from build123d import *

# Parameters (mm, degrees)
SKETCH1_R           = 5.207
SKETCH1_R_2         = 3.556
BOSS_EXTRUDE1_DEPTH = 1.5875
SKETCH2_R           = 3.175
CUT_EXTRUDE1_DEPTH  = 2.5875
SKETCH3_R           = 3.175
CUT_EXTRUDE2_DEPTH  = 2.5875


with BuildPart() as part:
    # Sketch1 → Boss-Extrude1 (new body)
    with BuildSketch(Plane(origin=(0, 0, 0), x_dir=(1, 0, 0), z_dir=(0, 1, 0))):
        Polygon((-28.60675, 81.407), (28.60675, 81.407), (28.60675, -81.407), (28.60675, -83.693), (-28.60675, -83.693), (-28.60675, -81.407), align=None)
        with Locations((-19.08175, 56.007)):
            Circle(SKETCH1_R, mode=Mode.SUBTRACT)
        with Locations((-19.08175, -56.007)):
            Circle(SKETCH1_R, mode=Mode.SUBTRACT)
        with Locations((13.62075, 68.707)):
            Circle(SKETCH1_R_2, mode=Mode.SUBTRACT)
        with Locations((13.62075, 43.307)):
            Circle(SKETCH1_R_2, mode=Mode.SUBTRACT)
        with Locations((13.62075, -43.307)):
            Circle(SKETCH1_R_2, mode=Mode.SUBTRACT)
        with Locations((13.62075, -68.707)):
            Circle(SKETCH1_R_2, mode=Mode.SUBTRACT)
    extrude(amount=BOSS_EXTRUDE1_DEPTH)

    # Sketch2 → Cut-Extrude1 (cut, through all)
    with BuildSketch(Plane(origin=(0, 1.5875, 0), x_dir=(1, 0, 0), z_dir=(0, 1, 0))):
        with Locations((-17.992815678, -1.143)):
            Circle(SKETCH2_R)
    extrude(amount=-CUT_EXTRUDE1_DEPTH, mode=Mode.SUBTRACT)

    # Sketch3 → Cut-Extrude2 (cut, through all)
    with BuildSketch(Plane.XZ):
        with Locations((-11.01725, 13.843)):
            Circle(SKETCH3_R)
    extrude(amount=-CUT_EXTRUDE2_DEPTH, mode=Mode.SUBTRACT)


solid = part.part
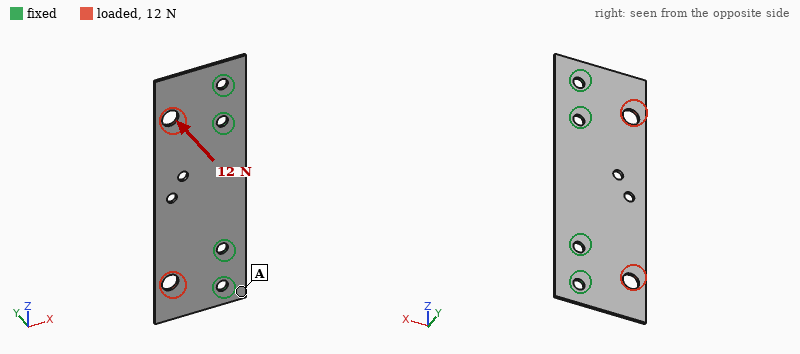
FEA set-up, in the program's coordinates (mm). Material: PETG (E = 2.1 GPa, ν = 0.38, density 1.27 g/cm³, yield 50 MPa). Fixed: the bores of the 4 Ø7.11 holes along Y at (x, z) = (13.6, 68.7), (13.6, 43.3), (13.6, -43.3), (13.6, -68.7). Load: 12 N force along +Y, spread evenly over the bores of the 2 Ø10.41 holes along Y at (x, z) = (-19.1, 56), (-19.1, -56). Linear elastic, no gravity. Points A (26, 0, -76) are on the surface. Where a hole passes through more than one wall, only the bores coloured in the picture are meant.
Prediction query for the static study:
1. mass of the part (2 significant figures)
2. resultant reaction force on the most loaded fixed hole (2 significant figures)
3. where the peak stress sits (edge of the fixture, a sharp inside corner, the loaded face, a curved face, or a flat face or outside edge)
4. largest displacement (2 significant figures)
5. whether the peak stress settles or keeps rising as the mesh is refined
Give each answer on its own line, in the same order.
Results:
18 g
3.3 N
edge of the fixture
2.0 mm
keeps rising
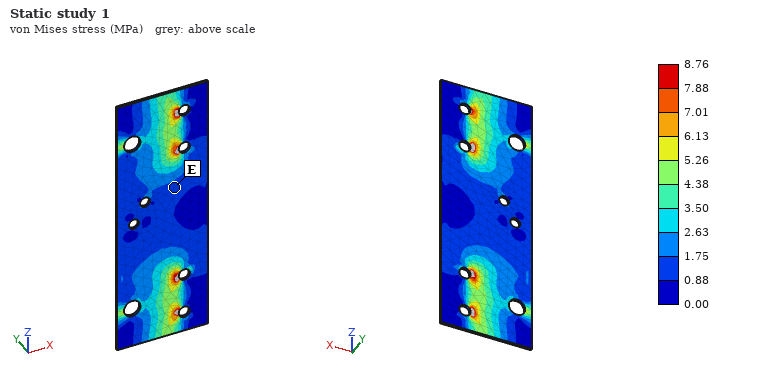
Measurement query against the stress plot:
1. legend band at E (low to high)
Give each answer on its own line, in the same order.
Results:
0.88 to 1.75 MPa
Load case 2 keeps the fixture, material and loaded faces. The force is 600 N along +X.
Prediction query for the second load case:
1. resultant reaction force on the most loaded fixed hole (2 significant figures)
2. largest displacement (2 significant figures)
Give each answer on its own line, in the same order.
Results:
160 N
0.16 mm
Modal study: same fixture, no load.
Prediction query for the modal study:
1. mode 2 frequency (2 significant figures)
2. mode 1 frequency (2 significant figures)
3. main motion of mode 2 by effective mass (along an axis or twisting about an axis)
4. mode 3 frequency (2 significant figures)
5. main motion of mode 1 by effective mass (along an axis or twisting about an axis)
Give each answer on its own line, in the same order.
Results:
250 Hz
170 Hz
twisting about X
270 Hz
along Y
